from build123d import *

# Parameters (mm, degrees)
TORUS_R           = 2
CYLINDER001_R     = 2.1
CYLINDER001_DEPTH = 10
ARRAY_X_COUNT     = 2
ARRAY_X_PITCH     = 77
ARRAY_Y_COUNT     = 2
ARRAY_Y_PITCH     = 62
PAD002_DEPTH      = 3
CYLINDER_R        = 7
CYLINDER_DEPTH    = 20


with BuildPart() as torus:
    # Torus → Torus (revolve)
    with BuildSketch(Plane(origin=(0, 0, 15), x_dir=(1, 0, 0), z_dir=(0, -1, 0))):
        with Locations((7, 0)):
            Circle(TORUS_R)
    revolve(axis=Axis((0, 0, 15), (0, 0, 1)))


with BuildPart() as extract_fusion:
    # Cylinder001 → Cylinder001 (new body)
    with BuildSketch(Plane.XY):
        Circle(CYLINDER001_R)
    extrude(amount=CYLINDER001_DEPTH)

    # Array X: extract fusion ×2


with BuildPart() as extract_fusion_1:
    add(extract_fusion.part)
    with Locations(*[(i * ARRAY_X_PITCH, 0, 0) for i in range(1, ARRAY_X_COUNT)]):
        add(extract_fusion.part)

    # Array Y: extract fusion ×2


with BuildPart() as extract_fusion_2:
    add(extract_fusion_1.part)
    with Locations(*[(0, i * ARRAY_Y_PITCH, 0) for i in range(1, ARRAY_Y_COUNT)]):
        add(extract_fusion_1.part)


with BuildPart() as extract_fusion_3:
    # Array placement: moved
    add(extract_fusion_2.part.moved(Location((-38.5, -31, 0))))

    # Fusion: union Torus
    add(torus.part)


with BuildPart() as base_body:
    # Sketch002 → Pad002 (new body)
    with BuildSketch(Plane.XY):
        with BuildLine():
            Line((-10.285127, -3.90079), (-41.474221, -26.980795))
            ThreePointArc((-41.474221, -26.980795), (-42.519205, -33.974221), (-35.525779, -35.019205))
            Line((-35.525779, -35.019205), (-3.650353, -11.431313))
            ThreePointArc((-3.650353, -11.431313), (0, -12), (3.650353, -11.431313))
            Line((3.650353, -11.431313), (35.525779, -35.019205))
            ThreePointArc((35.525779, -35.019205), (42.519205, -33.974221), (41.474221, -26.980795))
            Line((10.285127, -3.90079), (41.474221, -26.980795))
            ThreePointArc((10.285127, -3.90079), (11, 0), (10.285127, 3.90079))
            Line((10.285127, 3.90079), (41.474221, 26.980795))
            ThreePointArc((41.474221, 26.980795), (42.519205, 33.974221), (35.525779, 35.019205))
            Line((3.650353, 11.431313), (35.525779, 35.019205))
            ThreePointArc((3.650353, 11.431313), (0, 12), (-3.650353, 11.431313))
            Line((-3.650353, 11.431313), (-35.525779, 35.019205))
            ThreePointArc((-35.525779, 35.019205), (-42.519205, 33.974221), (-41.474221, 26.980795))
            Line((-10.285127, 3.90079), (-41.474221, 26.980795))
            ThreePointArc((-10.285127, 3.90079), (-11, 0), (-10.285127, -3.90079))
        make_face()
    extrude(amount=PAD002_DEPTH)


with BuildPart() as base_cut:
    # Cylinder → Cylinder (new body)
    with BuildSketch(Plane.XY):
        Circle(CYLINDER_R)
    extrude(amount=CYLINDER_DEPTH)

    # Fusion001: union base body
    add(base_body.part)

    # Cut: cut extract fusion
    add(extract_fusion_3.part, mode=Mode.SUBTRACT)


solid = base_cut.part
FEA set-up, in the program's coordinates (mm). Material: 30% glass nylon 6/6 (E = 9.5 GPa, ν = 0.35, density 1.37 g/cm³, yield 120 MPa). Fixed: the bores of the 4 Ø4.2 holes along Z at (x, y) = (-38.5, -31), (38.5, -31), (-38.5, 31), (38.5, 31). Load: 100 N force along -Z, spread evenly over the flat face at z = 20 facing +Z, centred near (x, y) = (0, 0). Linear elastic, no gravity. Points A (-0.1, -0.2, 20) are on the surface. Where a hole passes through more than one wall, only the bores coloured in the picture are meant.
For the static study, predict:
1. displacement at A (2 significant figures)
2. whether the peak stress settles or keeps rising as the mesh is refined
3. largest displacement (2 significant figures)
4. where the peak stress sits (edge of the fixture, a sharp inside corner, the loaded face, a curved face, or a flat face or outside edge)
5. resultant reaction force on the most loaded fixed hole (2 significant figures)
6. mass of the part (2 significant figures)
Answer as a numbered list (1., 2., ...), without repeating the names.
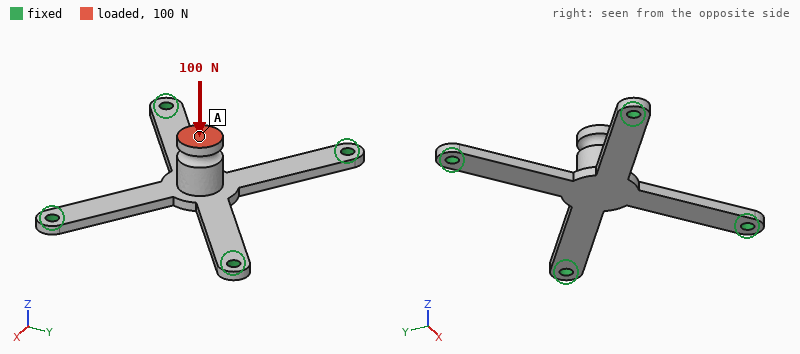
1. 0.71 mm
2. keeps rising
3. 0.71 mm
4. edge of the fixture
5. 26 N
6. 12 g
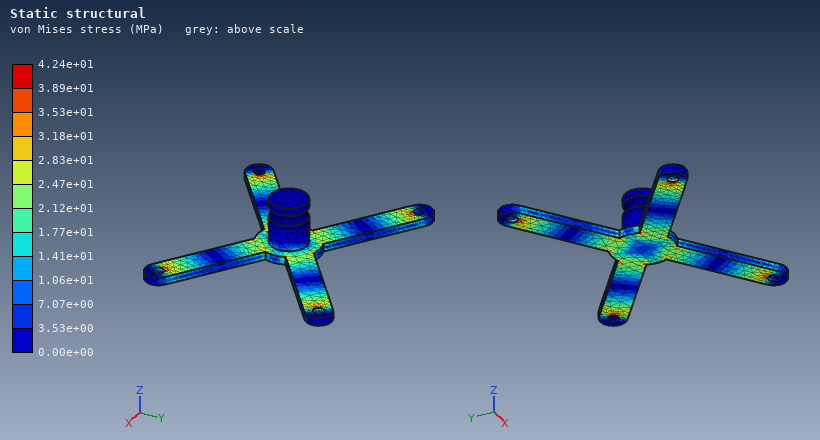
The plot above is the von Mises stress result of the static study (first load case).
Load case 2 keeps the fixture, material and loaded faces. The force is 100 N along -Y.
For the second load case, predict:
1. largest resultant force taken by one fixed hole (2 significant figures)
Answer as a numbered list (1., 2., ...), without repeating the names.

1. 43 N
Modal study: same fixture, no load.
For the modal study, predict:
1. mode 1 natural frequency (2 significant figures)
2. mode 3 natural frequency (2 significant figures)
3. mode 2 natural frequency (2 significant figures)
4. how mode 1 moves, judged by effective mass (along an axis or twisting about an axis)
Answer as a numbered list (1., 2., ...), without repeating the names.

1. 730 Hz
2. 1700 Hz
3. 1600 Hz
4. along Z
